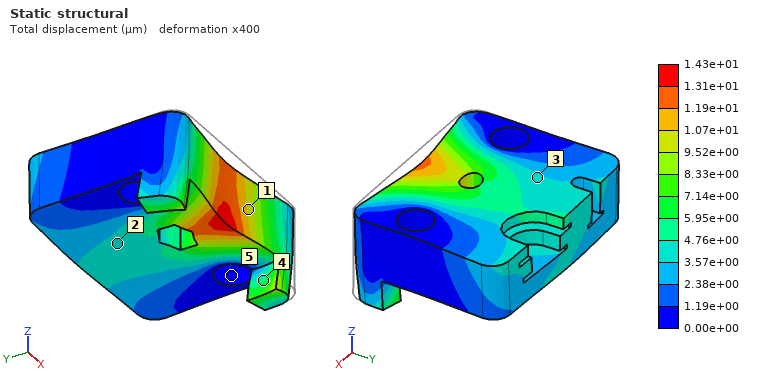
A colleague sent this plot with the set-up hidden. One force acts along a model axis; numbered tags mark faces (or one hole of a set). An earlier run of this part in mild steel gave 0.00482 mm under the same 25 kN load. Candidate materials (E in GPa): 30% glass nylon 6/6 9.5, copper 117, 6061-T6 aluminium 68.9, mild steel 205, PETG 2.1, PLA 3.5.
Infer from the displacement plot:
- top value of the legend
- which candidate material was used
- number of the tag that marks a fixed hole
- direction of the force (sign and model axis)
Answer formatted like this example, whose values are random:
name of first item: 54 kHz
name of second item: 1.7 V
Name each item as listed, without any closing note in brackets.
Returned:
top value of the legend: 1.43e+01 µm
which candidate material was used: 6061-T6 aluminium
number of the tag that marks a fixed hole: 5
direction of the force: +Y
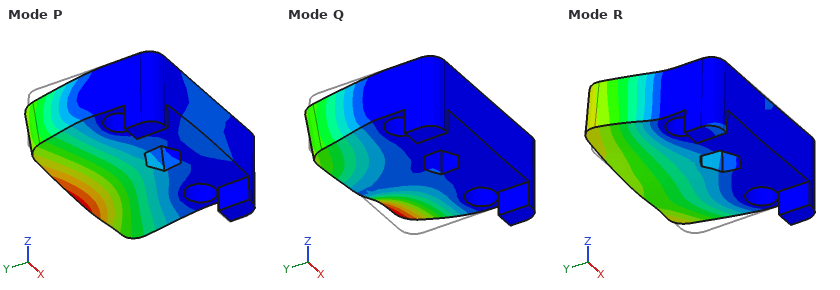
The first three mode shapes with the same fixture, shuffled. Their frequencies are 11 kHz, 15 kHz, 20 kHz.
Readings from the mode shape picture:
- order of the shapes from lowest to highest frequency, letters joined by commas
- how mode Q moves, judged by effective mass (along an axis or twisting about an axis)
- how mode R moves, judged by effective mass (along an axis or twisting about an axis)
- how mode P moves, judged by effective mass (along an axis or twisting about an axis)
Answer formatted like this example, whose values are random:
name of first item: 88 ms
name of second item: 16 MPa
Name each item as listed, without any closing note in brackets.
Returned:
order of the shapes from lowest to highest frequency, letters joined by commas: P, Q, R
how mode Q moves, judged by effective mass: twisting about Y
how mode R moves, judged by effective mass: along X
how mode P moves, judged by effective mass: along Z
